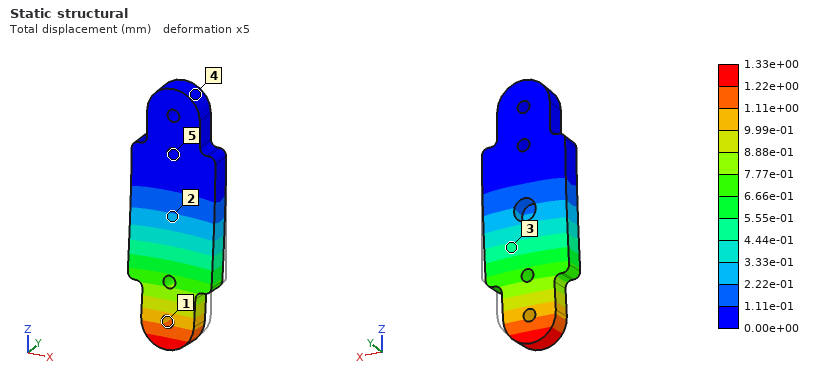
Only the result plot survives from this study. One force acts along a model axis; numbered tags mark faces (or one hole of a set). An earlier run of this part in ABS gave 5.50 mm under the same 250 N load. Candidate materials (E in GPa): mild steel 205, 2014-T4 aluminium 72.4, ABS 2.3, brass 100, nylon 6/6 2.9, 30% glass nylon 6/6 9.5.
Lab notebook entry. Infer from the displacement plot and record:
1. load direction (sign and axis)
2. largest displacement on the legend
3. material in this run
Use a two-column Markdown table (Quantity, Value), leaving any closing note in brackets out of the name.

| Quantity | Value |
|---|---|
| load direction | -Y |
| largest displacement on the legend | 1.33e+00 mm |
| material in this run | 30% glass nylon 6/6 |
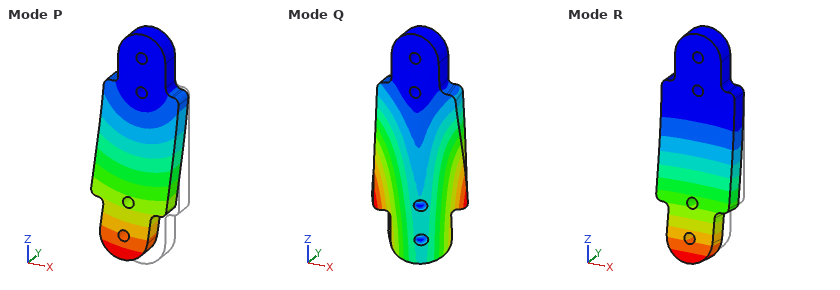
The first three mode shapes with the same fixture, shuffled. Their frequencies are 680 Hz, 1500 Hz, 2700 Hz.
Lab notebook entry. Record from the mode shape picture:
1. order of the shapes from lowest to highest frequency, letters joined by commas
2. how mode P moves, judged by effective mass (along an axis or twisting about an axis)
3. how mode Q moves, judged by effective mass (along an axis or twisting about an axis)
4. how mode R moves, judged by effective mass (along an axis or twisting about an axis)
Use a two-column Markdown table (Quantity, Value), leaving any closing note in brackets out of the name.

| Quantity | Value |
|---|---|
| order of the shapes from lowest to highest frequency, letters joined by commas | R, P, Q |
| how mode P moves, judged by effective mass | along X |
| how mode Q moves, judged by effective mass | twisting about Z |
| how mode R moves, judged by effective mass | along Y |
